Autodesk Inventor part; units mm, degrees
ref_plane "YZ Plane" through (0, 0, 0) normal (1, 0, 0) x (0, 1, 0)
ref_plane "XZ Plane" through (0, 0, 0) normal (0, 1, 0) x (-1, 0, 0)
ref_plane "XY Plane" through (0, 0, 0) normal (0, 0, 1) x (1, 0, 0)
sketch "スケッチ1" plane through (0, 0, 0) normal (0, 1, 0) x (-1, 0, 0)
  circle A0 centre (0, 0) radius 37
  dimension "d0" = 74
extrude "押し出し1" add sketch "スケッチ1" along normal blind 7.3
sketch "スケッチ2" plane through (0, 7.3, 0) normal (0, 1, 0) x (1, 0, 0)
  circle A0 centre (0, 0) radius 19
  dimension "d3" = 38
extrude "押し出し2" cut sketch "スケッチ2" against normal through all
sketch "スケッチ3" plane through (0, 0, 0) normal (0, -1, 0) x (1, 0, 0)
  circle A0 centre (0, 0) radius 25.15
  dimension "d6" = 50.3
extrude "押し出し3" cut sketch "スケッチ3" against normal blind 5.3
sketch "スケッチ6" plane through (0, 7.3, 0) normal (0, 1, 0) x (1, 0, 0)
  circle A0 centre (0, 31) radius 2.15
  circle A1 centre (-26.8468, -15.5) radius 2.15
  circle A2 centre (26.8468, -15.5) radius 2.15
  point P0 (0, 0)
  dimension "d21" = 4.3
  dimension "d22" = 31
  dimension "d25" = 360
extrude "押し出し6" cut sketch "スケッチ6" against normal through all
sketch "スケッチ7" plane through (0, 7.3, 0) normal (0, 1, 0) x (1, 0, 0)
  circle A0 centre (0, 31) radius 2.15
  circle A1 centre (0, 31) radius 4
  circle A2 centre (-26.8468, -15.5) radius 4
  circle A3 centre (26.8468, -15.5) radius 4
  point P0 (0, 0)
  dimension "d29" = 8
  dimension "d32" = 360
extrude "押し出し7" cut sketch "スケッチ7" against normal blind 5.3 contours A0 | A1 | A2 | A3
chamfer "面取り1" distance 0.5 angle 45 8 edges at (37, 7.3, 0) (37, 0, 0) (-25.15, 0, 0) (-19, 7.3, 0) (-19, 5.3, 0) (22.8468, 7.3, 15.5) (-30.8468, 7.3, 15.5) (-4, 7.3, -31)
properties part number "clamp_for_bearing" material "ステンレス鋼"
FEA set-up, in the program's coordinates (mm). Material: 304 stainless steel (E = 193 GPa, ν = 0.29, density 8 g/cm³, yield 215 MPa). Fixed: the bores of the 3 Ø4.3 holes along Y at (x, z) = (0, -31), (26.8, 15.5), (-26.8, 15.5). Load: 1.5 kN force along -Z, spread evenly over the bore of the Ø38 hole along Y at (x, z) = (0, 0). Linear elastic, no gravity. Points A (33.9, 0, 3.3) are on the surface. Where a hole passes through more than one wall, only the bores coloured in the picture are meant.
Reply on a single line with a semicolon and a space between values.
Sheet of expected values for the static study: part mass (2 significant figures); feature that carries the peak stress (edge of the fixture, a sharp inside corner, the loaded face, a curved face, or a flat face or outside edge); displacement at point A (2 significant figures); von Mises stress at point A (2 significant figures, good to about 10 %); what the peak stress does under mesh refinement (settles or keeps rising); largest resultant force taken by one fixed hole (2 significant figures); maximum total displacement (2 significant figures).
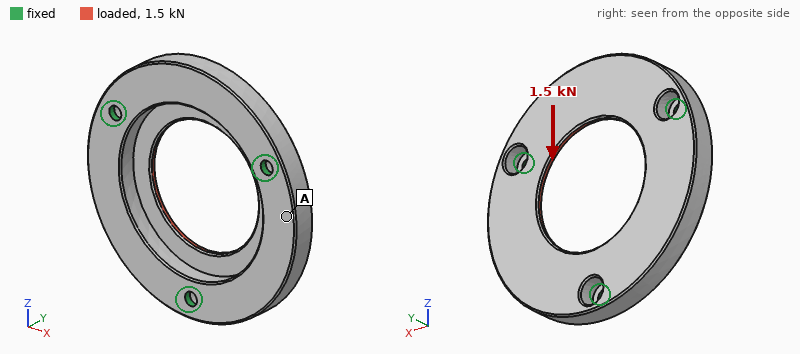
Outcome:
140 g; edge of the fixture; 2.9 µm; 7.9 MPa; keeps rising; 540 N; 9.6 µm
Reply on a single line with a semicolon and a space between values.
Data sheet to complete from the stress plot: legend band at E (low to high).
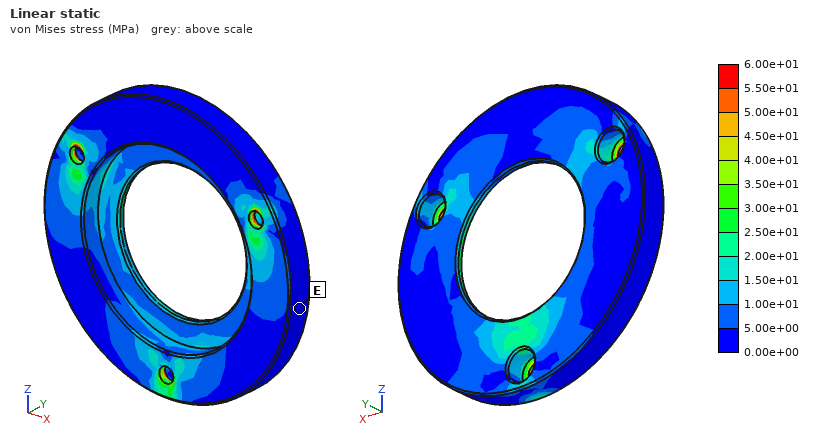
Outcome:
0.00e+00 to 5.00e+00 MPa
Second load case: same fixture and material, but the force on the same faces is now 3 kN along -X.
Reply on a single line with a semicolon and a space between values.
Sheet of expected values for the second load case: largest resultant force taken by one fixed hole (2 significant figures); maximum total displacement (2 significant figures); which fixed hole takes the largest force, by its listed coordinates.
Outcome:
1.1 kN; 17 µm; (0, -31)
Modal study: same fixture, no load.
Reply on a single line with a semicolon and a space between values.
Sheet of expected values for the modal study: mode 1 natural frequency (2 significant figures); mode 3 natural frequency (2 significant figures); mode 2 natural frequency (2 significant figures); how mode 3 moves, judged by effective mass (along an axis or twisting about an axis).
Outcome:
4400 Hz; 6700 Hz; 4400 Hz; along Y
